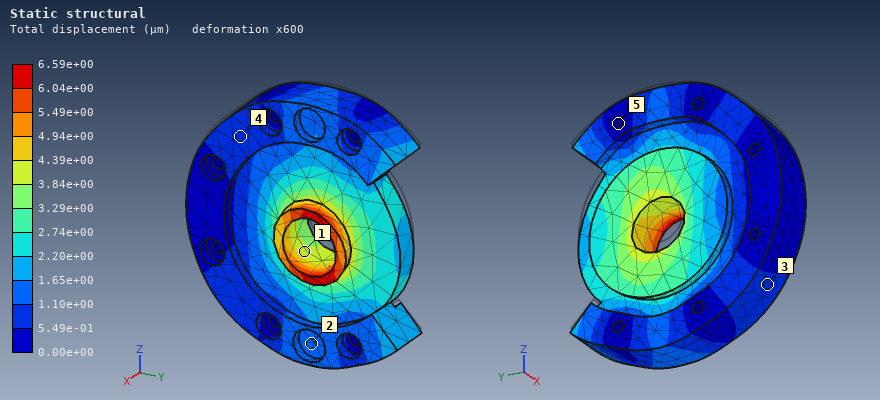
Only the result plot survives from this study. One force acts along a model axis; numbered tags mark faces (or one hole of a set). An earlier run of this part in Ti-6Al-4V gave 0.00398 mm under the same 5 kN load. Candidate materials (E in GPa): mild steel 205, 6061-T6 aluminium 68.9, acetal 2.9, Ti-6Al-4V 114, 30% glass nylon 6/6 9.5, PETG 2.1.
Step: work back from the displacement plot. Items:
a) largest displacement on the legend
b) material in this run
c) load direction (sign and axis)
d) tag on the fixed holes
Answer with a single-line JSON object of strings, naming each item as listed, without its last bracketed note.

{"largest displacement on the legend": "6.59e+00 µm", "material in this run": "6061-T6 aluminium", "load direction": "-Z", "tag on the fixed holes": "5"}
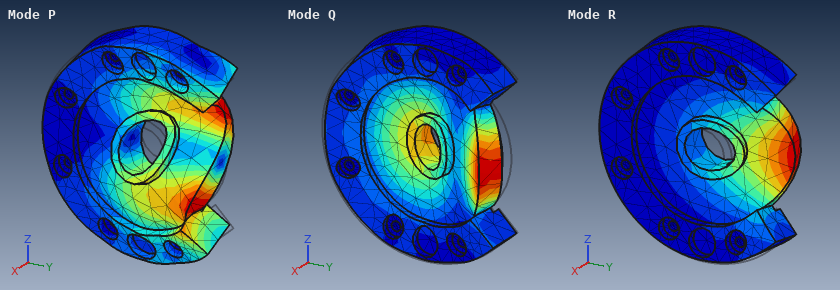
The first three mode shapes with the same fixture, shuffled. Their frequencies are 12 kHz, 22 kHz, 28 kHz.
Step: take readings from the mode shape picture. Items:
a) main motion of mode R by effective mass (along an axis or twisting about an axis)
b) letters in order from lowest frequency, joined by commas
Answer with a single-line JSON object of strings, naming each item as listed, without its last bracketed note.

{"main motion of mode R by effective mass": "along X", "letters in order from lowest frequency, joined by commas": "R, Q, P"}
